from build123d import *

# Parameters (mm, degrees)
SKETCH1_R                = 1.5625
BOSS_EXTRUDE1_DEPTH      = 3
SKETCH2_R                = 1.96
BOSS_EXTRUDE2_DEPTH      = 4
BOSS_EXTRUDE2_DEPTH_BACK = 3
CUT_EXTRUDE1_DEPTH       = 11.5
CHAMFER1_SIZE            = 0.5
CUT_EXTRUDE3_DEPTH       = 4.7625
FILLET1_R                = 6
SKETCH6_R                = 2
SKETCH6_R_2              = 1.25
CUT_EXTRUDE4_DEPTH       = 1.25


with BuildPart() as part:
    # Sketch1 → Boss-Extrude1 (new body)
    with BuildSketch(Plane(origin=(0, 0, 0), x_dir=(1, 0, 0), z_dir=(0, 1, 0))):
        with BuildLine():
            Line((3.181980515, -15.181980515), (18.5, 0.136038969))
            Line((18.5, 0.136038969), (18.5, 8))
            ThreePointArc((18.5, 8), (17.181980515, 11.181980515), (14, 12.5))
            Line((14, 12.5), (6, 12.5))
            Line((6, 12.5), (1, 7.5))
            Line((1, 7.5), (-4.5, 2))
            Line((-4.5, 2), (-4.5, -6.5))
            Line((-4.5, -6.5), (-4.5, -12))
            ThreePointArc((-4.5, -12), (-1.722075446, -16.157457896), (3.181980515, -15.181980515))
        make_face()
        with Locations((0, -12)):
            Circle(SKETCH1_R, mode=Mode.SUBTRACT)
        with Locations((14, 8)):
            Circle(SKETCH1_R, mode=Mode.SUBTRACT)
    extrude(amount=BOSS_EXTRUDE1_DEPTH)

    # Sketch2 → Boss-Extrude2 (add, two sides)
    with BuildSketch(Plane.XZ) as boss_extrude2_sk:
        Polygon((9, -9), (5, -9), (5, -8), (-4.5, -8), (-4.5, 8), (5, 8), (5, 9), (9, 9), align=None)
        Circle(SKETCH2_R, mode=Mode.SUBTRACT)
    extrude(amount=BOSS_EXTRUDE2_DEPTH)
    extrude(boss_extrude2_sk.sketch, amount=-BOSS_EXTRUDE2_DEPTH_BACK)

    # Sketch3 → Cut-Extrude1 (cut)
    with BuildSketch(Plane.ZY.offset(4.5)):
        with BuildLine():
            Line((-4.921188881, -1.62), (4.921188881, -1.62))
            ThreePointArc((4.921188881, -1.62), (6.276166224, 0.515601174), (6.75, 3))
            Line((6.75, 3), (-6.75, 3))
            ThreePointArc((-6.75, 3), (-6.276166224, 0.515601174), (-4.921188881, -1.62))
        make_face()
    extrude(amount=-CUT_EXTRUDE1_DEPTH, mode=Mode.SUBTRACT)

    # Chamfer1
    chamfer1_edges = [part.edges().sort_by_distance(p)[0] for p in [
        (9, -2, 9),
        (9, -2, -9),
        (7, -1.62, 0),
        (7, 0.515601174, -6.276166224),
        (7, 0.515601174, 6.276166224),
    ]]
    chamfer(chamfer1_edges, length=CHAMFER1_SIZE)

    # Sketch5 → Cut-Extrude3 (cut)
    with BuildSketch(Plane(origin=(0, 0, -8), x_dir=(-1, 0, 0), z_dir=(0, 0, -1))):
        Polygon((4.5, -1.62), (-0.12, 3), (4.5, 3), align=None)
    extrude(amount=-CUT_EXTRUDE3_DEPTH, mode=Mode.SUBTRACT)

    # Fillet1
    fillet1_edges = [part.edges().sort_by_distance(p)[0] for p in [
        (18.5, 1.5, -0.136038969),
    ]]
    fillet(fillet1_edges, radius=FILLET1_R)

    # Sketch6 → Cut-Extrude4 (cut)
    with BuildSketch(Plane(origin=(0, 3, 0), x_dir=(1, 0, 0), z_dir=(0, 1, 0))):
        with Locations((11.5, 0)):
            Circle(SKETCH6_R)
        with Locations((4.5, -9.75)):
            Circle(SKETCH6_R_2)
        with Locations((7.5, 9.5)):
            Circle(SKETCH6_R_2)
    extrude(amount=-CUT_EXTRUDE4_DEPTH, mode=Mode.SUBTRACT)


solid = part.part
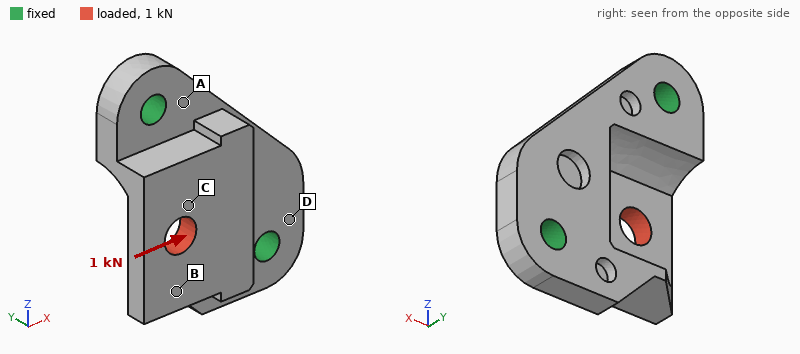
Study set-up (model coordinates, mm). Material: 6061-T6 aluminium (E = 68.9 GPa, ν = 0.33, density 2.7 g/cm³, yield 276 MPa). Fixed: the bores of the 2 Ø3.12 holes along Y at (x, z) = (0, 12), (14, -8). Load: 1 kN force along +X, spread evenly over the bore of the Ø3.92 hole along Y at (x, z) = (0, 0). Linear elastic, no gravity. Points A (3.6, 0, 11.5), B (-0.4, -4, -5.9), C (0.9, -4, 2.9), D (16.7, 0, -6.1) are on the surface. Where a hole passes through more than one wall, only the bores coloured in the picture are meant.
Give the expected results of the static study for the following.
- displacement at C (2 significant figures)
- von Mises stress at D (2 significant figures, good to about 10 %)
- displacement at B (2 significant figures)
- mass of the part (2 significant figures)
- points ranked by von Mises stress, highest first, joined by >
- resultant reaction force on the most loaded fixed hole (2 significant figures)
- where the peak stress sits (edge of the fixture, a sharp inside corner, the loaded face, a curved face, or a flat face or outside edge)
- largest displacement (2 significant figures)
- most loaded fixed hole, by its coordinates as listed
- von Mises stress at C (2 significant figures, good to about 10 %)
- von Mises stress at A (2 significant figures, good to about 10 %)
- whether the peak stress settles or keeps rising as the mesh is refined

34 µm
37 MPa
57 µm
4.2 g
A > C > D > B
610 N
edge of the fixture
79 µm
(0, 12)
62 MPa
89 MPa
keeps rising
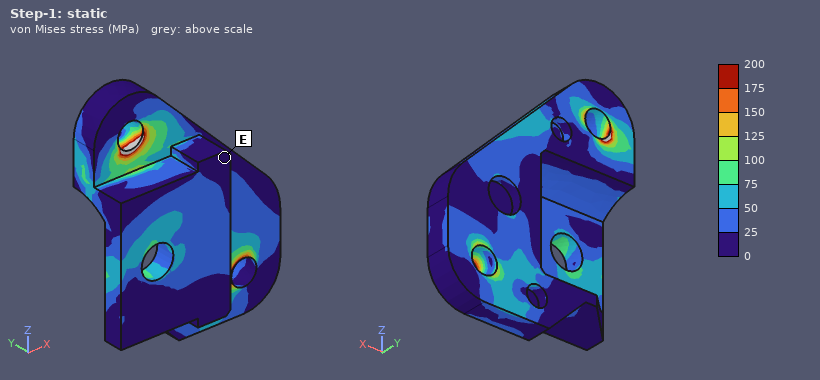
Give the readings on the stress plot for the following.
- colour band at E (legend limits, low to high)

0 to 25 MPa
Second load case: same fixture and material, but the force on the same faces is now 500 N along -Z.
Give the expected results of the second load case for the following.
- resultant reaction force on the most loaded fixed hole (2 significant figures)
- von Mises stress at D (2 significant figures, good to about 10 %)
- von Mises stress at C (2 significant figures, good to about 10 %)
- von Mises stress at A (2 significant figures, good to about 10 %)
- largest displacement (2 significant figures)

320 N
11 MPa
25 MPa
33 MPa
20 µm
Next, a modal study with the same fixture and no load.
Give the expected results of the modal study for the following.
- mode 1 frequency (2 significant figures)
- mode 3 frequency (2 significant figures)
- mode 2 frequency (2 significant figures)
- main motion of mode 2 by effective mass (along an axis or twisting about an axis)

13 kHz
28 kHz
24 kHz
along Y
